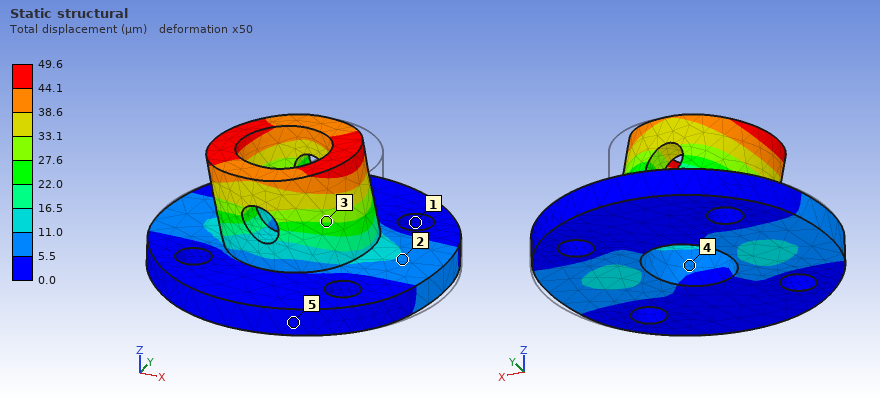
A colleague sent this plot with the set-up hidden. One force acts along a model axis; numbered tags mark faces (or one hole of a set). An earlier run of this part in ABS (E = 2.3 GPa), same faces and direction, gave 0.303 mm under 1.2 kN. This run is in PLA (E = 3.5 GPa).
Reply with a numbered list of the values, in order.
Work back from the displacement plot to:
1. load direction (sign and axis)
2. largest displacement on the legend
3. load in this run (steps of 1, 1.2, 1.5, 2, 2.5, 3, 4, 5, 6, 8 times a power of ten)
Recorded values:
1. -X
2. 49.6 µm
3. 300 N
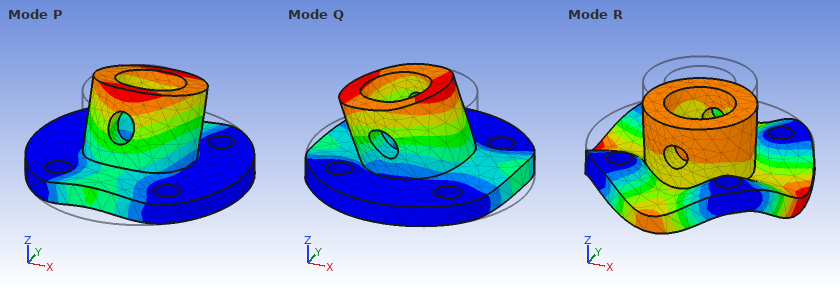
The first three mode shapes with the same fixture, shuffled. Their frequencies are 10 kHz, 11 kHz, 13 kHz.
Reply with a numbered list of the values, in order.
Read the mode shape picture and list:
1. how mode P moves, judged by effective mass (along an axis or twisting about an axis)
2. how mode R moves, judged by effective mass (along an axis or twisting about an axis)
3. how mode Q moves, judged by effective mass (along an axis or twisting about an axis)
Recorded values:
1. along Y
2. along Z
3. along X
